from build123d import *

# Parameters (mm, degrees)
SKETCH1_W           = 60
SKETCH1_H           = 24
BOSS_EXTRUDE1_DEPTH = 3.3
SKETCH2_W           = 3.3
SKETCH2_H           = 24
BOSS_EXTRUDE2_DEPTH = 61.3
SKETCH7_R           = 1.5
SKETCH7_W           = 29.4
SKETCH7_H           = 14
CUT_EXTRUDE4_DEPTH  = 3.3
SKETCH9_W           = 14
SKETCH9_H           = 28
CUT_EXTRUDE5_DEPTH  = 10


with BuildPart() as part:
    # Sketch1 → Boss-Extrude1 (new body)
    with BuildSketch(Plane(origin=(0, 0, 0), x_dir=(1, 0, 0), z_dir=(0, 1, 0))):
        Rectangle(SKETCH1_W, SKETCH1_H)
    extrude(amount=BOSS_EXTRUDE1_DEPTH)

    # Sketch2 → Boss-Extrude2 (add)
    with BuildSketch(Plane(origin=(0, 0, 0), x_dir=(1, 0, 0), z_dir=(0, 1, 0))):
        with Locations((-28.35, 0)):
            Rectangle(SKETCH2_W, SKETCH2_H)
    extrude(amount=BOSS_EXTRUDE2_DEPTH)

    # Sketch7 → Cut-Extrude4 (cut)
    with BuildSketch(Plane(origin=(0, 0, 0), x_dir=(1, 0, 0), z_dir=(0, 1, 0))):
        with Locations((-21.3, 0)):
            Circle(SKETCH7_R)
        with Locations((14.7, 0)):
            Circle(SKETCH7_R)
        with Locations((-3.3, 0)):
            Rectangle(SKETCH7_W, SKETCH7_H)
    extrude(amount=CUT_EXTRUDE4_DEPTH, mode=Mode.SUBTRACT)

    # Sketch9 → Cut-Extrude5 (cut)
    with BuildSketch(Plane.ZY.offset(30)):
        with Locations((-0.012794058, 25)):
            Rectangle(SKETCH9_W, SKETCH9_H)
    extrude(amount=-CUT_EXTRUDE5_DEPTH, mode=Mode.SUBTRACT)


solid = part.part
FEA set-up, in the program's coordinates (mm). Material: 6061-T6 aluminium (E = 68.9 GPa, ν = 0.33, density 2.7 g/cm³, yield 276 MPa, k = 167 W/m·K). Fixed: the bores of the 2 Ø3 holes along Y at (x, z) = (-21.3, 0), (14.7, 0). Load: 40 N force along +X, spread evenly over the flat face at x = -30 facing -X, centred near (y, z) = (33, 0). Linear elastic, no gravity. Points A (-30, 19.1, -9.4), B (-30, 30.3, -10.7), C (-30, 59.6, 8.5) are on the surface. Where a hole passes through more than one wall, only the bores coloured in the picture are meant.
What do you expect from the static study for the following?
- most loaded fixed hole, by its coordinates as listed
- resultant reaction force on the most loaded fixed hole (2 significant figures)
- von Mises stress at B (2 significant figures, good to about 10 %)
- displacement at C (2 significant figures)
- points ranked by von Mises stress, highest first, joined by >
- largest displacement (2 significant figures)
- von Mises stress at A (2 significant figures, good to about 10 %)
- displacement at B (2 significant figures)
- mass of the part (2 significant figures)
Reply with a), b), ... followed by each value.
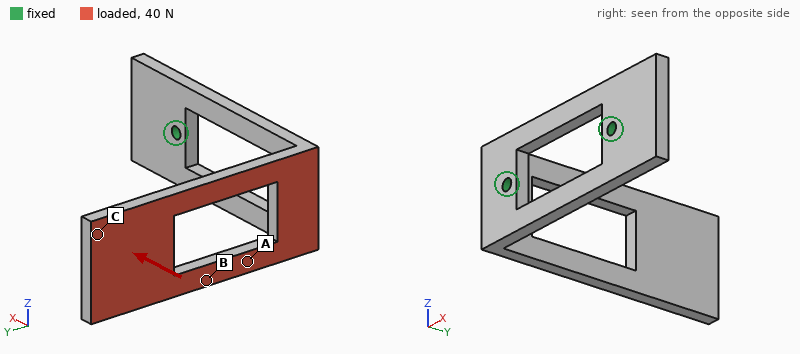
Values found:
a) (-21.3, 0)
b) 41 N
c) 23 MPa
d) 0.54 mm
e) A > B > C
f) 0.56 mm
g) 38 MPa
h) 0.19 mm
i) 18 g
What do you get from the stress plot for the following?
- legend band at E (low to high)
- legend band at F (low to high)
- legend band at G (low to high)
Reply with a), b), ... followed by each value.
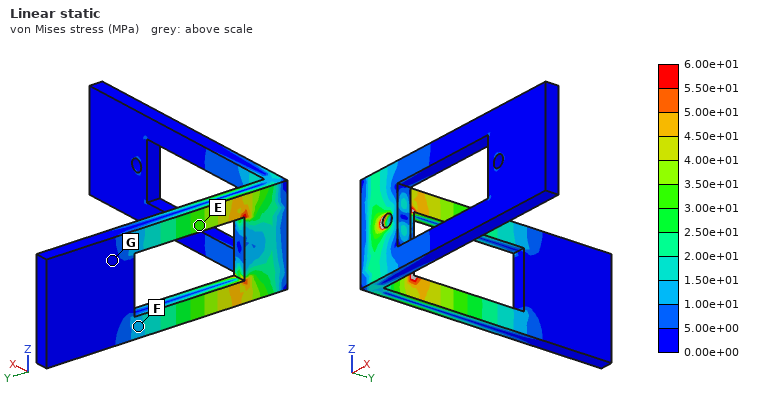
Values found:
a) 3.00e+01 to 3.50e+01 MPa
b) 1.00e+01 to 1.50e+01 MPa
c) 0.00e+00 to 5.00e+00 MPa
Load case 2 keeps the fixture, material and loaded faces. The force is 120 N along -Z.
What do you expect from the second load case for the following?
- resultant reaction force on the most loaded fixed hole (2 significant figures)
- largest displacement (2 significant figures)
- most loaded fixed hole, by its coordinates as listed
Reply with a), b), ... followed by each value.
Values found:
a) 130 N
b) 0.32 mm
c) (-21.3, 0)
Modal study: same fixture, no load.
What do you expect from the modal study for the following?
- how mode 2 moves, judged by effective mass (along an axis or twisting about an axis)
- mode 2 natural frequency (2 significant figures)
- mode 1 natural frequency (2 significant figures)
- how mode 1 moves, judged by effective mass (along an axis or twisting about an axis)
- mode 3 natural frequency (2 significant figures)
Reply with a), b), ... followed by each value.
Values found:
a) along Z
b) 1100 Hz
c) 510 Hz
d) along X
e) 2500 Hz
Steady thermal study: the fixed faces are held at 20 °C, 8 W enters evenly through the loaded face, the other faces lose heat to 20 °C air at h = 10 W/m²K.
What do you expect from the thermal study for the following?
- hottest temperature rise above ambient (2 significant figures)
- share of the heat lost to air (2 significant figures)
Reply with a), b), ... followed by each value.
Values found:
a) 39 K
b) 6.6 %
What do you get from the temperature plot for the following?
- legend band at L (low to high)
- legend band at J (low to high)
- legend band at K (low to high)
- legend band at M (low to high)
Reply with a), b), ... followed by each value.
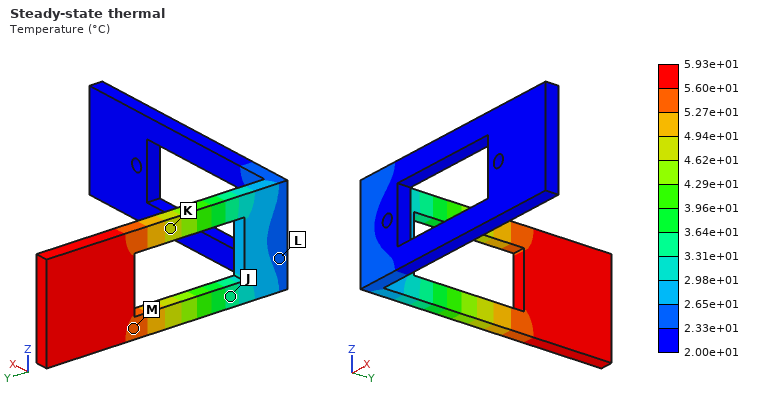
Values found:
a) 2.33e+01 to 2.65e+01 °C
b) 3.31e+01 to 3.64e+01 °C
c) 4.62e+01 to 4.94e+01 °C
d) 5.27e+01 to 5.60e+01 °C
